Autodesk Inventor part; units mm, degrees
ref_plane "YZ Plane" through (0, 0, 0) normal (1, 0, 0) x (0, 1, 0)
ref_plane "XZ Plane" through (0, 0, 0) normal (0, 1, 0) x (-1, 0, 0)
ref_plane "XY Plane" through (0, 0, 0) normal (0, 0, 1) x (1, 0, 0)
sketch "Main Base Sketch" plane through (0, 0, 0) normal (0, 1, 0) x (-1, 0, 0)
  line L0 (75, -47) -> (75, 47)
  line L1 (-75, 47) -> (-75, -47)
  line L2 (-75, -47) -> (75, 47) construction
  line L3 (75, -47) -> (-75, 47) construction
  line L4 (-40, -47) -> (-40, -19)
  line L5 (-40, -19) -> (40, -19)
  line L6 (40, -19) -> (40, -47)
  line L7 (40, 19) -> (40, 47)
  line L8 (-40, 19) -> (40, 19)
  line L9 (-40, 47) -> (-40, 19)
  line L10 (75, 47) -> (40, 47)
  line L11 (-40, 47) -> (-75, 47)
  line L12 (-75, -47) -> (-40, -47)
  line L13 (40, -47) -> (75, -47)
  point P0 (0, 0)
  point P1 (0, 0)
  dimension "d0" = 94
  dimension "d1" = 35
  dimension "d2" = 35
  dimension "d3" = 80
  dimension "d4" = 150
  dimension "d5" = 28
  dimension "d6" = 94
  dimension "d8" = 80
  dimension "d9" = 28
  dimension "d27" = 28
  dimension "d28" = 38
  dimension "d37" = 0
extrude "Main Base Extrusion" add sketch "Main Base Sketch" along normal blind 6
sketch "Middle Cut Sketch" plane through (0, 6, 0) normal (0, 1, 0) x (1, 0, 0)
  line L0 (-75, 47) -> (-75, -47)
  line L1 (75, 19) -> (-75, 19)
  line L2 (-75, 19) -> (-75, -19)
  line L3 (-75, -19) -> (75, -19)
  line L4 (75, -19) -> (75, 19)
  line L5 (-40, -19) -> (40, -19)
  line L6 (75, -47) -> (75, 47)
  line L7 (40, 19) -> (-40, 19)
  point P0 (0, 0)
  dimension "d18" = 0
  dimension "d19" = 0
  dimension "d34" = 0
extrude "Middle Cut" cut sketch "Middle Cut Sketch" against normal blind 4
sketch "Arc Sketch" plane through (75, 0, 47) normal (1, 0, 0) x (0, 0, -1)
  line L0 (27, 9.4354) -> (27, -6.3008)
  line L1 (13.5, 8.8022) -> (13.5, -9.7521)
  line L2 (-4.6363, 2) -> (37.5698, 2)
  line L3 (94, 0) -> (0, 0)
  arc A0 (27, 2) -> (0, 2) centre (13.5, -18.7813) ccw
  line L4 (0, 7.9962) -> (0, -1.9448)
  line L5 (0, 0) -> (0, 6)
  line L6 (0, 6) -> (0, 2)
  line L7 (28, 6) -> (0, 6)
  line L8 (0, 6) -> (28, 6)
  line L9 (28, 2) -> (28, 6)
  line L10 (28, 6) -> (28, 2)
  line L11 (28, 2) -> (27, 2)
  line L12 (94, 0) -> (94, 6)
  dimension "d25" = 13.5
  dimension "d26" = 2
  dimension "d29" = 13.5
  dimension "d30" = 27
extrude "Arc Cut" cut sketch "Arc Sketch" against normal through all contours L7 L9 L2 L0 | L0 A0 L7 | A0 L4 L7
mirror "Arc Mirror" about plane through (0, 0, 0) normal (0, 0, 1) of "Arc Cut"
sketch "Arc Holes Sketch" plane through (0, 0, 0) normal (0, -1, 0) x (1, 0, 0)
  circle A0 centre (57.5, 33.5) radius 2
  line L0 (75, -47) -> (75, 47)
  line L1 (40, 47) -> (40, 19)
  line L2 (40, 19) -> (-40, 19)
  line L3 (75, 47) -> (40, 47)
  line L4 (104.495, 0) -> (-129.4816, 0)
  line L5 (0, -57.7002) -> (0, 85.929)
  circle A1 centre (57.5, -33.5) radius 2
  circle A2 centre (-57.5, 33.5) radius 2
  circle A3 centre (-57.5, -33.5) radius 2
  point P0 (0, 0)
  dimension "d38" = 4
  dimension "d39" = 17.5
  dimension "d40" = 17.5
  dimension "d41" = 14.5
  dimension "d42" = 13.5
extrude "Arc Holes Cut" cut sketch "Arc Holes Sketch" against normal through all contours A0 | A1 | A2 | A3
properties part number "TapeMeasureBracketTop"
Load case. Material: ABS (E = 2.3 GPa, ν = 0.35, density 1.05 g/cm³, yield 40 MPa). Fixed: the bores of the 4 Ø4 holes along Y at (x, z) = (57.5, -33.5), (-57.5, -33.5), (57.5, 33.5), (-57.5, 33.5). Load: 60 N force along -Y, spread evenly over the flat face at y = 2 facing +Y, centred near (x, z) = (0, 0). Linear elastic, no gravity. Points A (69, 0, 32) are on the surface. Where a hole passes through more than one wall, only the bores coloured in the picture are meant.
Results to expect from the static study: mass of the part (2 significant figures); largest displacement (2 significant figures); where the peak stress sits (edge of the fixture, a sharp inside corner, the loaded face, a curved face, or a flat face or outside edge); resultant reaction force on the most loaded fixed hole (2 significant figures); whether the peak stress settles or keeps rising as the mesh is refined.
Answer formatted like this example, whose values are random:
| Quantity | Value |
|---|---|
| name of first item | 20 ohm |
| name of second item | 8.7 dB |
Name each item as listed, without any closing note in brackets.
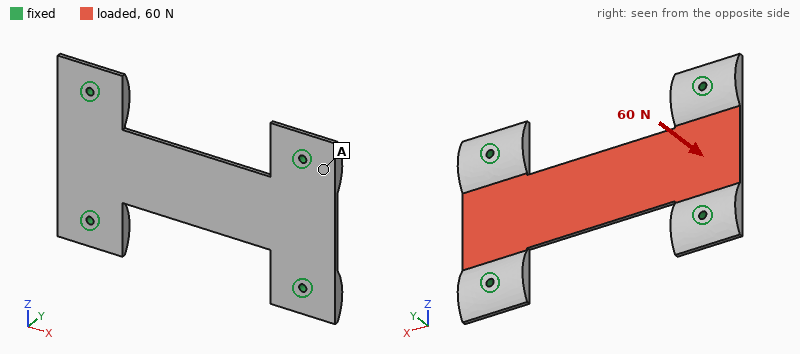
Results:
| Quantity | Value |
|---|---|
| mass of the part | 31 g |
| largest displacement | 1.7 mm |
| where the peak stress sits | a sharp inside corner |
| resultant reaction force on the most loaded fixed hole | 32 N |
| whether the peak stress settles or keeps rising as the mesh is refined | keeps rising |
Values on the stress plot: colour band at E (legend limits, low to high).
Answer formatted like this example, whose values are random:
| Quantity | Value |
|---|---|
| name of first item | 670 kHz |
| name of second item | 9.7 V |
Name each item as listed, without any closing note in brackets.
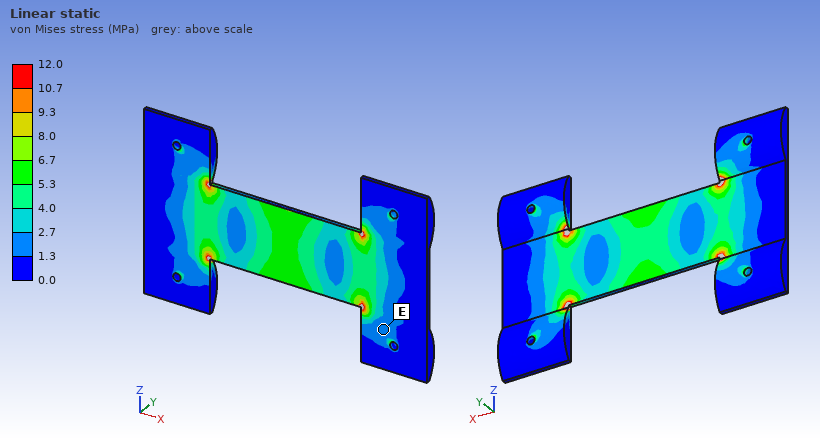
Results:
| Quantity | Value |
|---|---|
| colour band at E | 1.3 to 2.7 MPa |
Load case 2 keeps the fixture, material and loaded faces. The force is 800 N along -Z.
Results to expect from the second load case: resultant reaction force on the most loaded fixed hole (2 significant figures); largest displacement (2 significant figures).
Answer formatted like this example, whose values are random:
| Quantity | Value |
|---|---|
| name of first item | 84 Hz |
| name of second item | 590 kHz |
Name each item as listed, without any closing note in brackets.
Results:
| Quantity | Value |
|---|---|
| resultant reaction force on the most loaded fixed hole | 220 N |
| largest displacement | 0.92 mm |
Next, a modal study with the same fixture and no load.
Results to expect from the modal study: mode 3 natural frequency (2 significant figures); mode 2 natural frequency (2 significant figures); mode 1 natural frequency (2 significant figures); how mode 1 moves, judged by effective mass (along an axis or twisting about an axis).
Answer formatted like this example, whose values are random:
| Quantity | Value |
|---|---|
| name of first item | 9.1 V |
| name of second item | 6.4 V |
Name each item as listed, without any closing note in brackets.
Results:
| Quantity | Value |
|---|---|
| mode 3 natural frequency | 810 Hz |
| mode 2 natural frequency | 660 Hz |
| mode 1 natural frequency | 320 Hz |
| how mode 1 moves, judged by effective mass | along Y |
